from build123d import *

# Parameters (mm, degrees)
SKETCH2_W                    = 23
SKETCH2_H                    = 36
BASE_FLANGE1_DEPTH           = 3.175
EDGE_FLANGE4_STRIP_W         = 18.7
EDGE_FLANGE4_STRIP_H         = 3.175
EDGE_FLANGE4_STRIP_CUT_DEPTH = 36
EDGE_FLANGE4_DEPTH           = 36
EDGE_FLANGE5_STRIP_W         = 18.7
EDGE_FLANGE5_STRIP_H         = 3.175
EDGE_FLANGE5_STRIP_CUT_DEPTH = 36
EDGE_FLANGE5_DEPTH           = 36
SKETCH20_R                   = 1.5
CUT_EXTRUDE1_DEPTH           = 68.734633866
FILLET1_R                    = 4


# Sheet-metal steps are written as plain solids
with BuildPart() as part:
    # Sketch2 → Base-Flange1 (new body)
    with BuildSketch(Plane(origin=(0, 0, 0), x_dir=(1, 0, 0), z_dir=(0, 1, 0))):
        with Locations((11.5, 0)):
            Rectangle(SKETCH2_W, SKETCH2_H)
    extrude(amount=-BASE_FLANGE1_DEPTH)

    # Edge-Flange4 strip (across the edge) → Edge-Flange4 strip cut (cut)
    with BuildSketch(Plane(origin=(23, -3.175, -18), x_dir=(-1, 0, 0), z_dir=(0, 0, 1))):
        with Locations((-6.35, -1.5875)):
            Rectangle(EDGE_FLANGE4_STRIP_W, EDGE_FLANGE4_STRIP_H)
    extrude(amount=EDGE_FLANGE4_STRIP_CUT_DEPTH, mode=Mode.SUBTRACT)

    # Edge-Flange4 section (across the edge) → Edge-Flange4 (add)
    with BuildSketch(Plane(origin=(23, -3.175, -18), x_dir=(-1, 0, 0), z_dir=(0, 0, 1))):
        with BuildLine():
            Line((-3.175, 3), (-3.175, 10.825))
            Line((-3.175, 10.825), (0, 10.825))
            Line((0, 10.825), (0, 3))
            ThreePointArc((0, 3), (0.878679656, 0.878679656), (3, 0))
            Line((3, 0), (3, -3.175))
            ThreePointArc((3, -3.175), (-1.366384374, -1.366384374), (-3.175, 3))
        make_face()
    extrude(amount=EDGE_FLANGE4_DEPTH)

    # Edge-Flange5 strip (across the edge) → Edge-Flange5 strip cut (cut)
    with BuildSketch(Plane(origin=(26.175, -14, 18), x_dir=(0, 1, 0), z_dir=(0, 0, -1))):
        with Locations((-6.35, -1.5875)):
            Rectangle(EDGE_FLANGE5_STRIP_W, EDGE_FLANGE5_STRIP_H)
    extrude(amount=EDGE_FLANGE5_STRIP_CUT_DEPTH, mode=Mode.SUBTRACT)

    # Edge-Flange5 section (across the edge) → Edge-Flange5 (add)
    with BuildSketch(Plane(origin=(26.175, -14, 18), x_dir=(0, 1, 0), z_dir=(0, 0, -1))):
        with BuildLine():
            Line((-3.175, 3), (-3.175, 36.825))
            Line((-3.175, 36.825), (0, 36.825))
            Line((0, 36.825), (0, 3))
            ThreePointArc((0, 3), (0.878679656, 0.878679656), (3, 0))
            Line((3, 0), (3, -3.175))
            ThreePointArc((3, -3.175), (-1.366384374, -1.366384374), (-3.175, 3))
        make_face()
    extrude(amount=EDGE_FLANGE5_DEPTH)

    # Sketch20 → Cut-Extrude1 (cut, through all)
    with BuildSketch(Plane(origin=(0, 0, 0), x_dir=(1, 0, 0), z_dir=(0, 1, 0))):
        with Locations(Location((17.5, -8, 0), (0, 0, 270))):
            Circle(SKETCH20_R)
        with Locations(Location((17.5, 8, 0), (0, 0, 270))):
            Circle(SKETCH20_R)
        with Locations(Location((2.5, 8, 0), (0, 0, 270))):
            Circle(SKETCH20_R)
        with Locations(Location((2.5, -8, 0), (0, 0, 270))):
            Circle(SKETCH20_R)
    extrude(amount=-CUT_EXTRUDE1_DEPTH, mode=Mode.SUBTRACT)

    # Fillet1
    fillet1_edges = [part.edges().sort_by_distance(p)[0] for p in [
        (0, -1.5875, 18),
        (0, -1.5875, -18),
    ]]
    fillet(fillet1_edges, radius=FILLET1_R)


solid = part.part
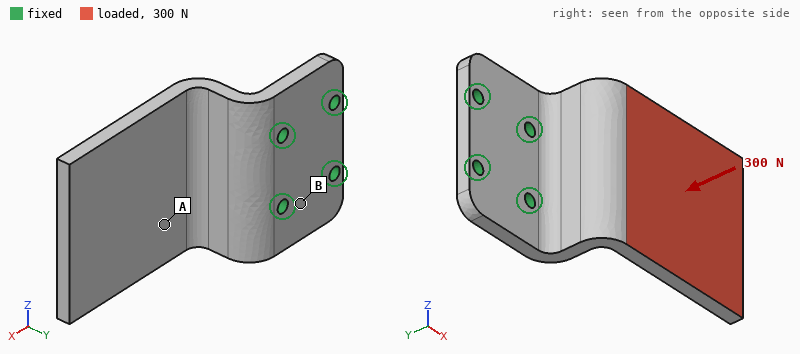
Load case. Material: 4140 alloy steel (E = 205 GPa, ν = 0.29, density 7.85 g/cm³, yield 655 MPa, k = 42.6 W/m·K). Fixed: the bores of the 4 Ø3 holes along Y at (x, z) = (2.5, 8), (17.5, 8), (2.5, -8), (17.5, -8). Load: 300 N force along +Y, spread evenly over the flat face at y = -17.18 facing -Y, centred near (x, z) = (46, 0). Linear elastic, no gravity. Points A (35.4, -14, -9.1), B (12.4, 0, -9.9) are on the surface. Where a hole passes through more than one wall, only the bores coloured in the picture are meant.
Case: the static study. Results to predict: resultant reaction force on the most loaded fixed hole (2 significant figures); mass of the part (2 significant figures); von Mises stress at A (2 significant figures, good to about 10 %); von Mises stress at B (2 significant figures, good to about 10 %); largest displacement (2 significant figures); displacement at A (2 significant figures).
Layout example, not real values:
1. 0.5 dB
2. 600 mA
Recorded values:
1. 240 N
2. 65 g
3. 52 MPa
4. 17 MPa
5. 0.36 mm
6. 0.10 mm
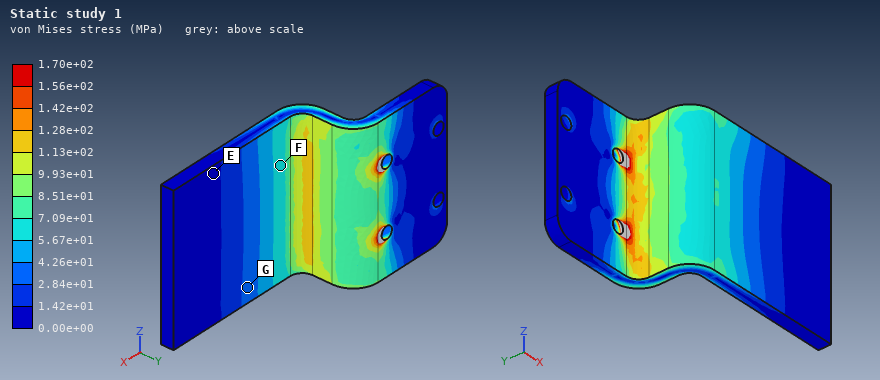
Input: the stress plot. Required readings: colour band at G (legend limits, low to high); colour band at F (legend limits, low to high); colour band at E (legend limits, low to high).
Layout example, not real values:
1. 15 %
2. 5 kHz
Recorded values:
1. 2.84e+01 to 4.26e+01 MPa
2. 5.67e+01 to 7.09e+01 MPa
3. 0.00e+00 to 1.42e+01 MPa
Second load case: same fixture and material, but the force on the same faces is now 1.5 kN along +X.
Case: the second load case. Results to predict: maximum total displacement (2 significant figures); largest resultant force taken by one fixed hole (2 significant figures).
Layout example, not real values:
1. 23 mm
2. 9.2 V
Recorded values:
1. 0.69 mm
2. 680 N
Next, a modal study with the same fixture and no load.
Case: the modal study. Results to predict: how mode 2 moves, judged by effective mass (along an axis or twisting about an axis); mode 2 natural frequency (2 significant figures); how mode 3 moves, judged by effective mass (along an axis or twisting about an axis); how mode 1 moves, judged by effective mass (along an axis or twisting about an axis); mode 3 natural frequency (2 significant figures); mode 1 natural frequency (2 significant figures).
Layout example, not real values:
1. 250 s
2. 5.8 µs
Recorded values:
1. along Z
2. 2400 Hz
3. along X
4. along Y
5. 4200 Hz
6. 980 Hz
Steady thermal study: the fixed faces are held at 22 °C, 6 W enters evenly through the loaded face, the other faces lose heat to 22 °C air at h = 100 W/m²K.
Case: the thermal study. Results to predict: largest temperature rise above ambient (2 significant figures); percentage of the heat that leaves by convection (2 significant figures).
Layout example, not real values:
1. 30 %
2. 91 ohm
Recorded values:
1. 21 K
2. 65 %
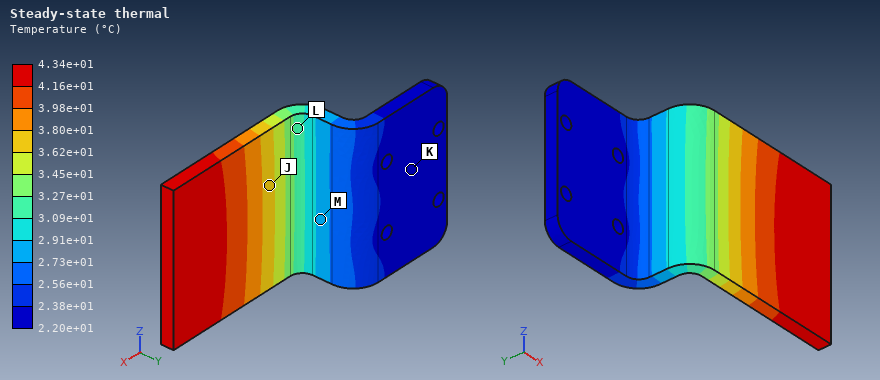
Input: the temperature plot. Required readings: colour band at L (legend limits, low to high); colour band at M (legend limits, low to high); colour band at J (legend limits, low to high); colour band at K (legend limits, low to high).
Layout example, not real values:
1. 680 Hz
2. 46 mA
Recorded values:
1. 3.09e+01 to 3.27e+01 °C
2. 2.73e+01 to 2.91e+01 °C
3. 3.62e+01 to 3.80e+01 °C
4. 2.20e+01 to 2.38e+01 °C
